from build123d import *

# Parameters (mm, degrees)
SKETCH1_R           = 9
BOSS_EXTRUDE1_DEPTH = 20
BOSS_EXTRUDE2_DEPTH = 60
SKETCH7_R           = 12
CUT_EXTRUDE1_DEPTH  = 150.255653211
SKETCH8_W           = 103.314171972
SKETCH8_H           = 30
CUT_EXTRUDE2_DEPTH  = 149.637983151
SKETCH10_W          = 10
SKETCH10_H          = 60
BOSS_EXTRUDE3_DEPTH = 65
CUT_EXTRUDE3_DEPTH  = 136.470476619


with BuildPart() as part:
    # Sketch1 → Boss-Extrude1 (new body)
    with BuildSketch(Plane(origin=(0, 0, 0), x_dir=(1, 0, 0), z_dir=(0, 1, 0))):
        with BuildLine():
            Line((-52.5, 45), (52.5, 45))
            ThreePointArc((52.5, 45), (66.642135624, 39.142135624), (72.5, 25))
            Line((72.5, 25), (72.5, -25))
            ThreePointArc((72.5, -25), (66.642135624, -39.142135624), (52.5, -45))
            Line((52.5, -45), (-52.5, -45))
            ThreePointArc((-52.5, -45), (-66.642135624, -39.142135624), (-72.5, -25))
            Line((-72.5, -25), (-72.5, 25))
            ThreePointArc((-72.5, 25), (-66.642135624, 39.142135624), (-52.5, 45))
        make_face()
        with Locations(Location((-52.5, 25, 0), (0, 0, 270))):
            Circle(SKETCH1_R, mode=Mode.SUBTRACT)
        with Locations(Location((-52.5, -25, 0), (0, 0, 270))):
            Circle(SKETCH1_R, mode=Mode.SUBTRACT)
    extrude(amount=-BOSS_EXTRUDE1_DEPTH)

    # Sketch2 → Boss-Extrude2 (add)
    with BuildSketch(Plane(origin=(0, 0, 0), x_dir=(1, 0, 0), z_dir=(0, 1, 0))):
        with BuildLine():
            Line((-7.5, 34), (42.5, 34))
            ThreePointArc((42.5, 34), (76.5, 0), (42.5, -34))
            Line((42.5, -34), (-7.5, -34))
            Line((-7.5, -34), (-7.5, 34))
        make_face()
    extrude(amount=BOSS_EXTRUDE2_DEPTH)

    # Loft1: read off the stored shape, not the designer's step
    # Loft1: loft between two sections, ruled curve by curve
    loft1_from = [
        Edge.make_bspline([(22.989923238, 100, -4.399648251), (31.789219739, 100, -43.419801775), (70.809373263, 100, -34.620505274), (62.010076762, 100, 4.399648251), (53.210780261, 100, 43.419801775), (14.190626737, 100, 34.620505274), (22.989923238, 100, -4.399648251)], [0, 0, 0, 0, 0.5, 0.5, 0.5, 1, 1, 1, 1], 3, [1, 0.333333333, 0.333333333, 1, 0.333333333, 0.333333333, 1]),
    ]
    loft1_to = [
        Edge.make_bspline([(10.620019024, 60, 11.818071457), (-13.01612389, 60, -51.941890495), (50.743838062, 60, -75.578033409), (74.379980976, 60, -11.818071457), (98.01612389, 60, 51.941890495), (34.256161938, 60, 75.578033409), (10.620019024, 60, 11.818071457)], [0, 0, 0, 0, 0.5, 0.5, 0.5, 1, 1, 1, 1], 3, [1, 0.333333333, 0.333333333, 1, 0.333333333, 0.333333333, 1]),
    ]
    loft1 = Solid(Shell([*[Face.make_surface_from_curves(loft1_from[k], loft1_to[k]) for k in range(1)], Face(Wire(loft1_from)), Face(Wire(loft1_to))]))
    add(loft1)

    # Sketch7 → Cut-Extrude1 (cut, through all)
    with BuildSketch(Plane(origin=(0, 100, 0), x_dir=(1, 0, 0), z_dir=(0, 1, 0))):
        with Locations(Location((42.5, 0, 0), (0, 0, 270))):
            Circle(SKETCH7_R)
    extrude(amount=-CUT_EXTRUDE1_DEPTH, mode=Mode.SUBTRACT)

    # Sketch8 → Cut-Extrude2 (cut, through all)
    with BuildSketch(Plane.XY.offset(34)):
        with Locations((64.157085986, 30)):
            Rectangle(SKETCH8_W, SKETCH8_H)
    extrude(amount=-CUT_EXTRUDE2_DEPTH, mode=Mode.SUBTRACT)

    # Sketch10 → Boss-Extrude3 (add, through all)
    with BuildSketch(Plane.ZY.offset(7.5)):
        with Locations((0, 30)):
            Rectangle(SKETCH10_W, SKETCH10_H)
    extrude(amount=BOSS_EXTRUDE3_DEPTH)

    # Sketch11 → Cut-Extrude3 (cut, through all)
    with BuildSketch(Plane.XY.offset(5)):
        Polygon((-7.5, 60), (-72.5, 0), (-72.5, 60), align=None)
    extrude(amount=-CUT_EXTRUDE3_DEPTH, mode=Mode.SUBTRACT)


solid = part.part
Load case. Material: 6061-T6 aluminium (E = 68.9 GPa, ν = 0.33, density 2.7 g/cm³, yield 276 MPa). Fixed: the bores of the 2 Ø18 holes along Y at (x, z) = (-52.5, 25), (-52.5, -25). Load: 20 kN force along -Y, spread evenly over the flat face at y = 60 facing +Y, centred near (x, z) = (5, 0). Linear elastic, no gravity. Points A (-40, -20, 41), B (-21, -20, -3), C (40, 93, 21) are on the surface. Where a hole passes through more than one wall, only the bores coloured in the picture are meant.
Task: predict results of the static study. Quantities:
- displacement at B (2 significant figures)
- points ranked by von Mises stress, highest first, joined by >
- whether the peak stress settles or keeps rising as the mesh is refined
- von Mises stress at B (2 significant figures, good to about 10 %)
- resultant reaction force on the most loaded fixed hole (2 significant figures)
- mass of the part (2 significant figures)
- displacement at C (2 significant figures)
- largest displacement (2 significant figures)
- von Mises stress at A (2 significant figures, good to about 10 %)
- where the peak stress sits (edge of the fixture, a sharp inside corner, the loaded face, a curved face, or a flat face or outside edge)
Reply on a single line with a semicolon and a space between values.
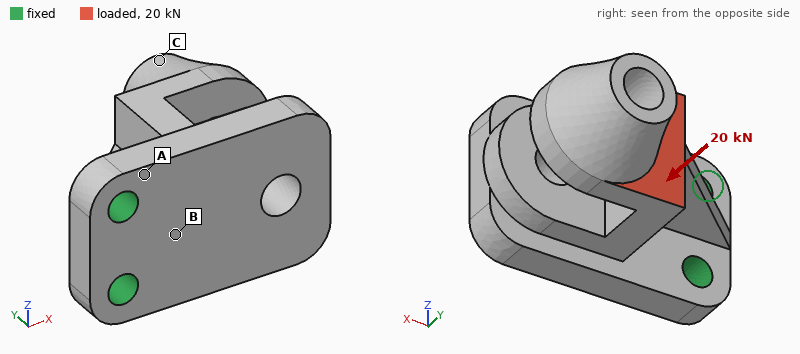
0.093 mm; A > B > C; keeps rising; 40 MPa; 10 kN; 1.4 kg; 0.53 mm; 0.61 mm; 85 MPa; edge of the fixture
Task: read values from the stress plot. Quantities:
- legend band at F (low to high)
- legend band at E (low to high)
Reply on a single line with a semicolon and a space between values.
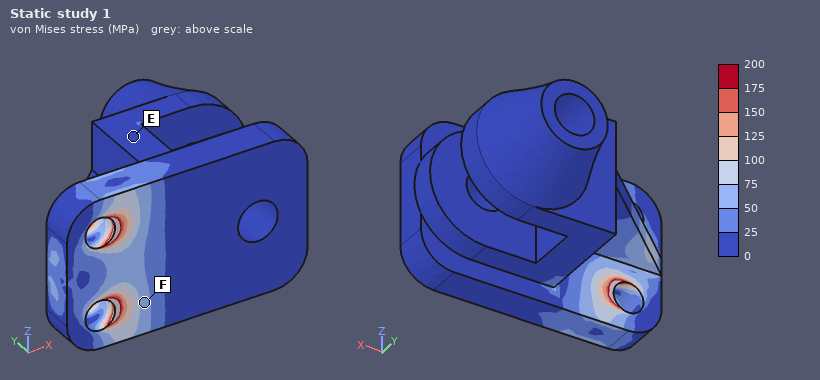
50 to 75 MPa; 0 to 25 MPa
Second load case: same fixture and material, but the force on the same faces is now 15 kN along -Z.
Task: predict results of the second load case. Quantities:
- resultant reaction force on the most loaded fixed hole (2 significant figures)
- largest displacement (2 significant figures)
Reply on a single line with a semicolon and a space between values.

23 kN; 0.55 mm
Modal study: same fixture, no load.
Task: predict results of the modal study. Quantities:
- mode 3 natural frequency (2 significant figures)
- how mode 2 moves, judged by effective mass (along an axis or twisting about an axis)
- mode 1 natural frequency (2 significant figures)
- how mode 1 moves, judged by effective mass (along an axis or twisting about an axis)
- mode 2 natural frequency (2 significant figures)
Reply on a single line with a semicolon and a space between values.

2100 Hz; along Z; 790 Hz; along Y; 1200 Hz
